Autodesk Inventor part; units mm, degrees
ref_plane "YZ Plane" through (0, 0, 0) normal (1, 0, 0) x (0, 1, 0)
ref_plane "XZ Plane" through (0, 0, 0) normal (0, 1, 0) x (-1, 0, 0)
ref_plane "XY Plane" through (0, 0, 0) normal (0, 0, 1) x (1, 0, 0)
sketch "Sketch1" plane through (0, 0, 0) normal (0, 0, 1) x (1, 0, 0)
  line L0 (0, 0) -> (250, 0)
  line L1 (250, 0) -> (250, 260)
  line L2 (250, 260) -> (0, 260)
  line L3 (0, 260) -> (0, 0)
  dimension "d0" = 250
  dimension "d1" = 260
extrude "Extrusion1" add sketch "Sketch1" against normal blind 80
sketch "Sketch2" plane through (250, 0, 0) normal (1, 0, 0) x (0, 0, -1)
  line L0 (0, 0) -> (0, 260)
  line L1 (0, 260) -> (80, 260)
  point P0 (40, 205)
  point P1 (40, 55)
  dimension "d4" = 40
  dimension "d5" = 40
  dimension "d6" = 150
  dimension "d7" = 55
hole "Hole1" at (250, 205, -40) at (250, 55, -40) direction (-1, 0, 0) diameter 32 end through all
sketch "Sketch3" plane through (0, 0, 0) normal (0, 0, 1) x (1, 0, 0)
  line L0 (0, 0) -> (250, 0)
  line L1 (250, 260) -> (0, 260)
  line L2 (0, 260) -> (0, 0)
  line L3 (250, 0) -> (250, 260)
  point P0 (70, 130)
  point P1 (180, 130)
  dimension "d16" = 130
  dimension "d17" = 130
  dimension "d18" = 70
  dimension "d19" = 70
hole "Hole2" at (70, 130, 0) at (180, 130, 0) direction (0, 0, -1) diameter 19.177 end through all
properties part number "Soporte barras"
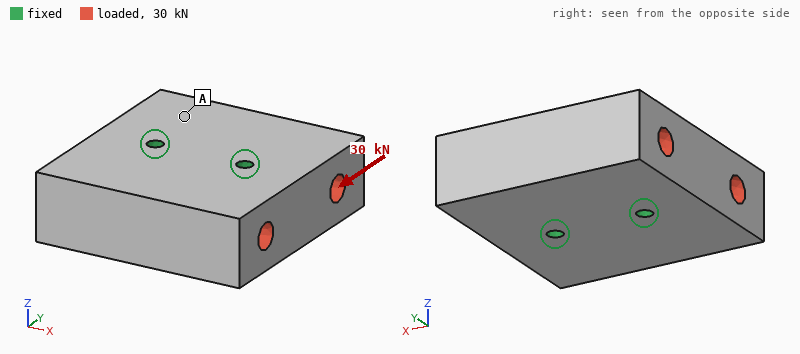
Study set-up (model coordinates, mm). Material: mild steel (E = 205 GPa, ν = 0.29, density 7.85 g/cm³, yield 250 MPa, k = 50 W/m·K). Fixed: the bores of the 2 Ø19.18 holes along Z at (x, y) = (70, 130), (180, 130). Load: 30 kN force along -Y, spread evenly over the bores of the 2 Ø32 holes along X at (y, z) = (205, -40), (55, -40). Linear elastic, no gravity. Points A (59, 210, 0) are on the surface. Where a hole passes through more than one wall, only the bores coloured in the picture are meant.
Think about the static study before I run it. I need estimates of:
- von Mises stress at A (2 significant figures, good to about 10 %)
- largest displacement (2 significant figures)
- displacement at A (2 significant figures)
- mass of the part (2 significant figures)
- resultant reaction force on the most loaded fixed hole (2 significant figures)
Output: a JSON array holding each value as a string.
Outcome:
["0.61 MPa", "0.75 µm", "0.52 µm", "37 kg", "15 kN"]
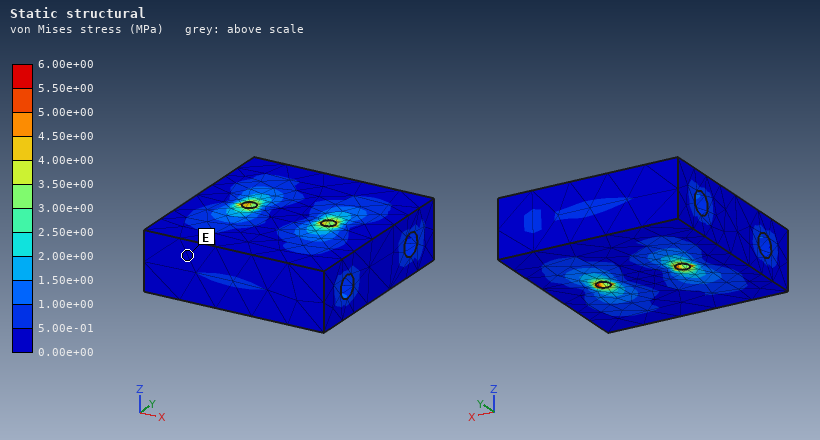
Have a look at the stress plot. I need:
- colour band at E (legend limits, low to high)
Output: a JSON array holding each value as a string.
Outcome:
["0.00e+00 to 5.00e-01 MPa"]
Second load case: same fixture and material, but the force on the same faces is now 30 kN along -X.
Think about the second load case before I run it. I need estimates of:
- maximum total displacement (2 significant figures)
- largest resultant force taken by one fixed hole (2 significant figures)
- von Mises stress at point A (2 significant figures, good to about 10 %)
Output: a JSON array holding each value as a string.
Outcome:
["1.3 µm", "15 kN", "0.84 MPa"]
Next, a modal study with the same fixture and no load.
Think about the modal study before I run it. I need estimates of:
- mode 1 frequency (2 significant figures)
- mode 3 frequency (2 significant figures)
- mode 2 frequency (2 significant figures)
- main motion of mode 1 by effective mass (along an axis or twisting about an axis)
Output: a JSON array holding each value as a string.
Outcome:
["2200 Hz", "3000 Hz", "3000 Hz", "twisting about X"]
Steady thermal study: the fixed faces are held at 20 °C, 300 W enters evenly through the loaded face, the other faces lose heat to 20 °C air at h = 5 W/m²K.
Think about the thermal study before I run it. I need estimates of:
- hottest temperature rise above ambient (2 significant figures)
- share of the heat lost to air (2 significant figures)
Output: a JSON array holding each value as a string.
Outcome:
["18 K", "4.6 %"]
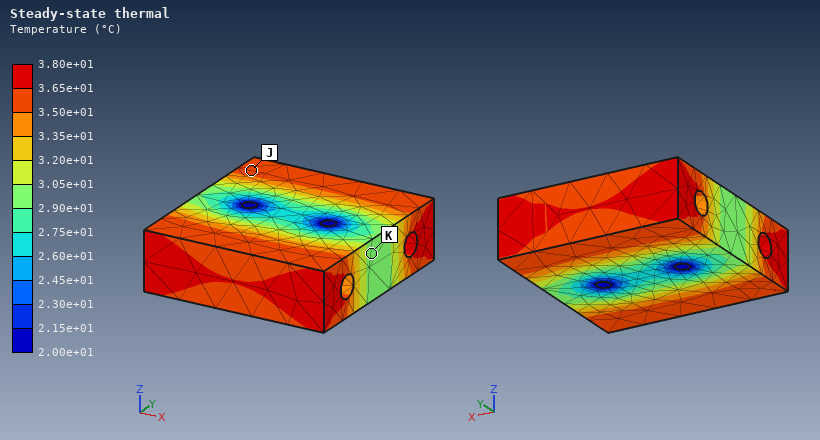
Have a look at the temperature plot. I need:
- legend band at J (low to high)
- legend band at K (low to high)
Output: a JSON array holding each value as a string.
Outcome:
["3.50e+01 to 3.65e+01 °C", "2.90e+01 to 3.05e+01 °C"]
